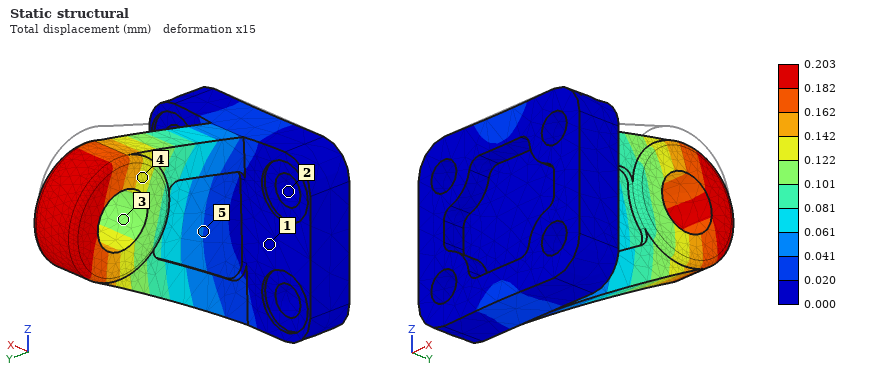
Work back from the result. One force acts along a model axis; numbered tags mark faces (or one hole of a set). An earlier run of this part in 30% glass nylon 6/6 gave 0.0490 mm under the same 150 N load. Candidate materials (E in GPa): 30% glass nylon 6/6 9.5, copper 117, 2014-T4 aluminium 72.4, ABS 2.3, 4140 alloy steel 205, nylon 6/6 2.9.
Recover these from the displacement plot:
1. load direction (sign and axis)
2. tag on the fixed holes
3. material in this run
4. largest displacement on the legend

-Z
2
ABS
0.203 mm
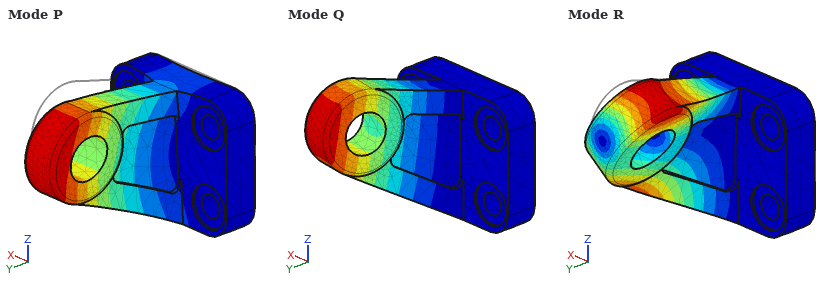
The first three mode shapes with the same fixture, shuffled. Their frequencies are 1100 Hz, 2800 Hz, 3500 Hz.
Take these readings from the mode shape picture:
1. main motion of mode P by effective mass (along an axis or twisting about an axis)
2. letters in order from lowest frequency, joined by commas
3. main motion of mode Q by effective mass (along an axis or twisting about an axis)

along Z
Q, P, R
along X
